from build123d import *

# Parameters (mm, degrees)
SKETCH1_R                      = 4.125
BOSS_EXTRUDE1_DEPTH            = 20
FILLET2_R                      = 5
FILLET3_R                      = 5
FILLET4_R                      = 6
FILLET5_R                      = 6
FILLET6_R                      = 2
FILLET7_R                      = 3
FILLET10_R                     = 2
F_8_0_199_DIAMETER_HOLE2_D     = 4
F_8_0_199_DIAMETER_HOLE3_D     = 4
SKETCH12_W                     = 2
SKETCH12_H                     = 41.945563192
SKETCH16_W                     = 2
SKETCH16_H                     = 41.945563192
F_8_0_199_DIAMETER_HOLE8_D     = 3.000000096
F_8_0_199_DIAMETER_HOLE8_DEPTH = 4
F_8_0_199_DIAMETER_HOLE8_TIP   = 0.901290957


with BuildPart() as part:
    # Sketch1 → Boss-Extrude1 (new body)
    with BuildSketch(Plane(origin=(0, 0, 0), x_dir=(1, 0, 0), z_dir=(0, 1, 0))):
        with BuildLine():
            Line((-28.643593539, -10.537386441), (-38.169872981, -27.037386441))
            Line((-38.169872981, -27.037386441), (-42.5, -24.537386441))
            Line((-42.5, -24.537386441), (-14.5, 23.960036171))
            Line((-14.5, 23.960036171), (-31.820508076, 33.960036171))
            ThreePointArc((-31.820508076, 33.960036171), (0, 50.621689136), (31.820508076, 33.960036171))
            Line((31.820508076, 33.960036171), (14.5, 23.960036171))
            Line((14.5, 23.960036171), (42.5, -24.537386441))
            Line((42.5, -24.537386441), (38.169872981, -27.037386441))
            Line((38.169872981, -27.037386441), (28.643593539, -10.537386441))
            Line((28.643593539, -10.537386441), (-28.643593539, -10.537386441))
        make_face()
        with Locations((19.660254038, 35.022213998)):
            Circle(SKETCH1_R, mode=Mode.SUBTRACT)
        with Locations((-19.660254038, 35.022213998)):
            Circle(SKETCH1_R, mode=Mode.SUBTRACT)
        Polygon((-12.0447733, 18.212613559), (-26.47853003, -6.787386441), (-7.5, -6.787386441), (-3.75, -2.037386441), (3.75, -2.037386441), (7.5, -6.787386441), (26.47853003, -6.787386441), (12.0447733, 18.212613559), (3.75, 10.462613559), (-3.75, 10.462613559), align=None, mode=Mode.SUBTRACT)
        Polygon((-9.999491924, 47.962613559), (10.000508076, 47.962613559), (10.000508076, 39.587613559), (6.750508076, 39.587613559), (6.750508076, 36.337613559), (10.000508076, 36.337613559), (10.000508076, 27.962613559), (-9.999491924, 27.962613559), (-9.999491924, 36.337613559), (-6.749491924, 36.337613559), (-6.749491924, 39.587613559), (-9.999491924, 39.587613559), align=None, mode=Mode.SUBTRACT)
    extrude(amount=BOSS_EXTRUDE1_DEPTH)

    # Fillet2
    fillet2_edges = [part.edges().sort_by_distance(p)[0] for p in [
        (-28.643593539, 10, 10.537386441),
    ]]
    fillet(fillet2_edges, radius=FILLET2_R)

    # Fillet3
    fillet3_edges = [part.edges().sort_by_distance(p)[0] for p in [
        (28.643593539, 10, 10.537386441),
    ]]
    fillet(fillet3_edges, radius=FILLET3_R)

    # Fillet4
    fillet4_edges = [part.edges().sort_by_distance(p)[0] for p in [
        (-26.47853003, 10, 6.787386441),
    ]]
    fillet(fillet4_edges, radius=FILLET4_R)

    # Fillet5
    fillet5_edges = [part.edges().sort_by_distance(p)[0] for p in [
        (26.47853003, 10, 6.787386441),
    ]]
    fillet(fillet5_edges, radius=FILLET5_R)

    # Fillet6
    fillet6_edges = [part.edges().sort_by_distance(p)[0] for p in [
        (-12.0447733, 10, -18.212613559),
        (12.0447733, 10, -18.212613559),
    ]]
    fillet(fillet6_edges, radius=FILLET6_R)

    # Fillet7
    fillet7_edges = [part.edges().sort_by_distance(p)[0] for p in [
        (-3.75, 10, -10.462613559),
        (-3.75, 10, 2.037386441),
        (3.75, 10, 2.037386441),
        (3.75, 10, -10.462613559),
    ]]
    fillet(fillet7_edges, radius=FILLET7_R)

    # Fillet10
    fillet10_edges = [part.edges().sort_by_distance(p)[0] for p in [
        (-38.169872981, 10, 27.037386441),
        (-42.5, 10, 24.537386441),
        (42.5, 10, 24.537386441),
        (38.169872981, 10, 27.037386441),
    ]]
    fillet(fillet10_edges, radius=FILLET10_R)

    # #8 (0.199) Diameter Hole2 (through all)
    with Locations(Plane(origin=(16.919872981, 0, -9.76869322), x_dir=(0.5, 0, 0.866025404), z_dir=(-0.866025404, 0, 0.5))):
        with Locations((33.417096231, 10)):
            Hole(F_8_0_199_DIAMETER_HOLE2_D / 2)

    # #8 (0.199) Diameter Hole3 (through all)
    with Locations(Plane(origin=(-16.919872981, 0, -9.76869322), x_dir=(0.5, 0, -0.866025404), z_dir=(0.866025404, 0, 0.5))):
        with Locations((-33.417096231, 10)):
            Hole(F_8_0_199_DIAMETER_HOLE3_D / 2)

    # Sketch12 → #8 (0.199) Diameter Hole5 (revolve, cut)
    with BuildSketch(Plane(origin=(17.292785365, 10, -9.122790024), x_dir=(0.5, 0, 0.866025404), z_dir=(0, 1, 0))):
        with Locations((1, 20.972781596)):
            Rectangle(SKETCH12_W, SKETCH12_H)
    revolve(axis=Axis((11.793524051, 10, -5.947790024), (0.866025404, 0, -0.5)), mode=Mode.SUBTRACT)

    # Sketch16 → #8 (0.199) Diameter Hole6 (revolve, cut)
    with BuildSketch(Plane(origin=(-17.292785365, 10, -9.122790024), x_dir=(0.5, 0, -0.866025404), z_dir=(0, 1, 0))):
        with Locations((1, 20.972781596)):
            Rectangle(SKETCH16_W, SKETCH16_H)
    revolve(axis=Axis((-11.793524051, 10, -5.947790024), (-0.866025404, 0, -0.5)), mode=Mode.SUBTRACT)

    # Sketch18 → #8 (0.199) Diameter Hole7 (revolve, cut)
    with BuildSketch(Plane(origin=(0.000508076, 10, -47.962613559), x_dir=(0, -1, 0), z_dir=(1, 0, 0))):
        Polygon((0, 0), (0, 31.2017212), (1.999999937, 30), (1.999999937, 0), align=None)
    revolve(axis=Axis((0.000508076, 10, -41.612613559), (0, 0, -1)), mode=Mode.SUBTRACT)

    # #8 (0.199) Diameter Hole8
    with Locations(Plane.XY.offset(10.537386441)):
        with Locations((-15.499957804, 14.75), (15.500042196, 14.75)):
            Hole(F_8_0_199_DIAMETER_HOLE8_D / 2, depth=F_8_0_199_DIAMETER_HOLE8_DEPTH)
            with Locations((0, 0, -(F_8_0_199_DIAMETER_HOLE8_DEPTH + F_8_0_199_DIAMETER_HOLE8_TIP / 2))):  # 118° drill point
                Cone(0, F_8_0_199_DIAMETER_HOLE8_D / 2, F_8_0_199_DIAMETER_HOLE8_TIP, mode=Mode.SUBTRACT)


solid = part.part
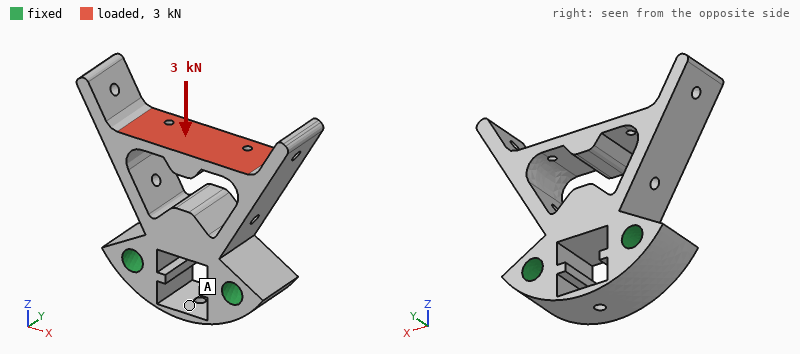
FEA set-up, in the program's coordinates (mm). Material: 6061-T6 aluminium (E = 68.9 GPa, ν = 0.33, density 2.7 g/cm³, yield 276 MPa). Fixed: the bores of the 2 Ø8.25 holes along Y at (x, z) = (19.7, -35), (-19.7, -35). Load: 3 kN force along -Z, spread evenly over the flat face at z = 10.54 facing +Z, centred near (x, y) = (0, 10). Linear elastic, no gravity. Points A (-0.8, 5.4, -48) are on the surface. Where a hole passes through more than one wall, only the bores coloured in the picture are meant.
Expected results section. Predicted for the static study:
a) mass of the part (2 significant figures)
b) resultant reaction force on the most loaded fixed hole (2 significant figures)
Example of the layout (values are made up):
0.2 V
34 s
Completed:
99 g
1.5 kN
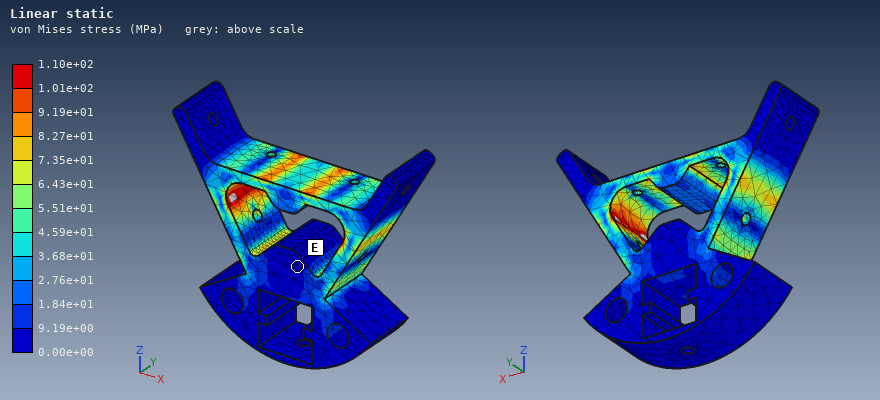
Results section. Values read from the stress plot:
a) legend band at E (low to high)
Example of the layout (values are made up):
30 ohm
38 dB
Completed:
0.00e+00 to 9.19e+00 MPa
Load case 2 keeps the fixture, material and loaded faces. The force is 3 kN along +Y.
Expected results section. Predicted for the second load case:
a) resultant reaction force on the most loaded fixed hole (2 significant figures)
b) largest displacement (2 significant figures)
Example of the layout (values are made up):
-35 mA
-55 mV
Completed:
1.5 kN
0.35 mm
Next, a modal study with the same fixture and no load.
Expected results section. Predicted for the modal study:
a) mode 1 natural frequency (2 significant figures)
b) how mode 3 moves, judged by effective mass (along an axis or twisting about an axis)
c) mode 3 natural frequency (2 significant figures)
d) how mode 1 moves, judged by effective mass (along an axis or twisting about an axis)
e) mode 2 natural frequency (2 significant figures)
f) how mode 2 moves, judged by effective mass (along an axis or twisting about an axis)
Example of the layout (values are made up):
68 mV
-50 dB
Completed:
1600 Hz
twisting about Z
3800 Hz
along X
3000 Hz
along Y
